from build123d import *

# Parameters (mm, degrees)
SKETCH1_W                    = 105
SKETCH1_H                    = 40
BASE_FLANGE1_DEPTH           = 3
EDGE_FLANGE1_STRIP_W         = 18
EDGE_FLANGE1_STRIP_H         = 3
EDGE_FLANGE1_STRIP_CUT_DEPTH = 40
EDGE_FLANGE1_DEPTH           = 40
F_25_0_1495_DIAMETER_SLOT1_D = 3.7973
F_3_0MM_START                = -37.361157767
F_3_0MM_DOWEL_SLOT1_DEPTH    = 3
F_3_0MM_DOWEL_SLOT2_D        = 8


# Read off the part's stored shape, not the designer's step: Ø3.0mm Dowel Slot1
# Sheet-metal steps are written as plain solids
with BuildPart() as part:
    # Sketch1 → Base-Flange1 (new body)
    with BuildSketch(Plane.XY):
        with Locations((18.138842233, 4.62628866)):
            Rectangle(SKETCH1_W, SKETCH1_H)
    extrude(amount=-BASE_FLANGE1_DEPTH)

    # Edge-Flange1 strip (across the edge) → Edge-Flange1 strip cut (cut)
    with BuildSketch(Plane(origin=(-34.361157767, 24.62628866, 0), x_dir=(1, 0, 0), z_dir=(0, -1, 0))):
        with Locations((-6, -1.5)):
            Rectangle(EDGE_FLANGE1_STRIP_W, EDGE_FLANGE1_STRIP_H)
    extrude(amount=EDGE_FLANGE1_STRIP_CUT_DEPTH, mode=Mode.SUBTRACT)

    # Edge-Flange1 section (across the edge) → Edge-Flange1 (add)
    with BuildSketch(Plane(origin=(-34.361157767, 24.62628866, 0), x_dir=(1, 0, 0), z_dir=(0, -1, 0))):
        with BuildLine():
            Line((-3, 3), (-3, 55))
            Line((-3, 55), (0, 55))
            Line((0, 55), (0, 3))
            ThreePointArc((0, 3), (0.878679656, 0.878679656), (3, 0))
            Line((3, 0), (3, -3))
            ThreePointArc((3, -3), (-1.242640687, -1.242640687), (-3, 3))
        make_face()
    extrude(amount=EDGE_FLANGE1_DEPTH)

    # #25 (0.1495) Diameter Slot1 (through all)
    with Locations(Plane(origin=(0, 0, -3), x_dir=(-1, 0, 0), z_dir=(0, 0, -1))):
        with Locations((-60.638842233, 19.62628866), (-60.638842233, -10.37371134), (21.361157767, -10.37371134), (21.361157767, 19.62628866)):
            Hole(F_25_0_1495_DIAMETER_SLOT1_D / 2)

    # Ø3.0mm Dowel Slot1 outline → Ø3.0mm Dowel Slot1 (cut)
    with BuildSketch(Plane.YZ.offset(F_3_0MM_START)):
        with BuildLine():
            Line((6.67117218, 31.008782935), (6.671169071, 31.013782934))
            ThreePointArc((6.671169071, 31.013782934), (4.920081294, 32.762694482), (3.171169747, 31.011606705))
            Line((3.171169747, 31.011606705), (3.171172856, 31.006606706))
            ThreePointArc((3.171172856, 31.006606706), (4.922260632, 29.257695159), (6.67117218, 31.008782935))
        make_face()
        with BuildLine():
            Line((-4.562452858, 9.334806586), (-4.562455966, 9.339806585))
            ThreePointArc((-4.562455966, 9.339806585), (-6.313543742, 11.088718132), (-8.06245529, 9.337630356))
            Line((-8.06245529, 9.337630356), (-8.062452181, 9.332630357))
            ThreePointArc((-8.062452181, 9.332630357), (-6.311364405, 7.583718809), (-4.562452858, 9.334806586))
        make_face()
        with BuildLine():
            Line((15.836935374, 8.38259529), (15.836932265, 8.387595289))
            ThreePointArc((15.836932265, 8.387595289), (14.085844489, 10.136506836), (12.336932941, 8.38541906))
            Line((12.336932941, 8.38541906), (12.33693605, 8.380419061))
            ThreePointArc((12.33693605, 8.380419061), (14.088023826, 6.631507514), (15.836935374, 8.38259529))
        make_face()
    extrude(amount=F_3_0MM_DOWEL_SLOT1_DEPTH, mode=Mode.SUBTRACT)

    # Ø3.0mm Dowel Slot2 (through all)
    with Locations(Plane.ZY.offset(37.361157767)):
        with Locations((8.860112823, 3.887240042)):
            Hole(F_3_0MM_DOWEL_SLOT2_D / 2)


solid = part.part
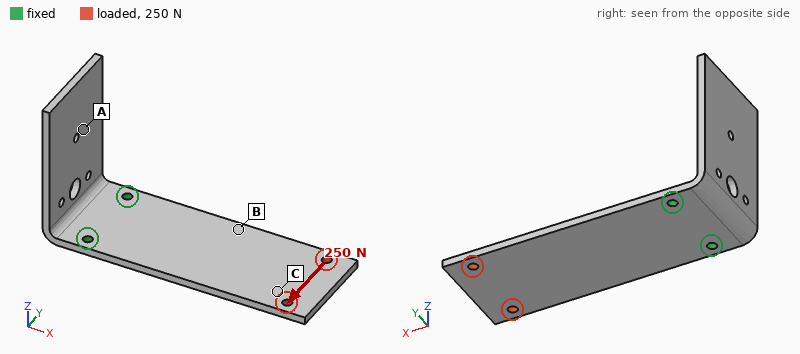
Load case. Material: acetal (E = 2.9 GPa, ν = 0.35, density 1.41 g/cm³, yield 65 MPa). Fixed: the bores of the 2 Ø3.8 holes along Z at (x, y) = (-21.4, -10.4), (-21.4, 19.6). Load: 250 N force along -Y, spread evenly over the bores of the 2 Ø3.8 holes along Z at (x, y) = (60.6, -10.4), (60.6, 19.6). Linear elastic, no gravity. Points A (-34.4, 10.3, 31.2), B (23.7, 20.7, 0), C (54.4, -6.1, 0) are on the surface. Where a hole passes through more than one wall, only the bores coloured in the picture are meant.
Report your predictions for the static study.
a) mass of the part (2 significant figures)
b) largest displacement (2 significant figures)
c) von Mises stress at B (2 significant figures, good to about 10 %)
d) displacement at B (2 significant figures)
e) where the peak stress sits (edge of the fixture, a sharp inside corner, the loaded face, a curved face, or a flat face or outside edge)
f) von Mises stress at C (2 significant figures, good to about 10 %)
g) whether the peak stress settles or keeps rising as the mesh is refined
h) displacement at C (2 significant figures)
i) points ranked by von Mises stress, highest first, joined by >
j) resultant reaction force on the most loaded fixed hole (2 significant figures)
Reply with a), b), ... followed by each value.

a) 27 g
b) 1.4 mm
c) 9.4 MPa
d) 0.54 mm
e) edge of the fixture
f) 4.7 MPa
g) keeps rising
h) 1.1 mm
i) B > C > A
j) 670 N
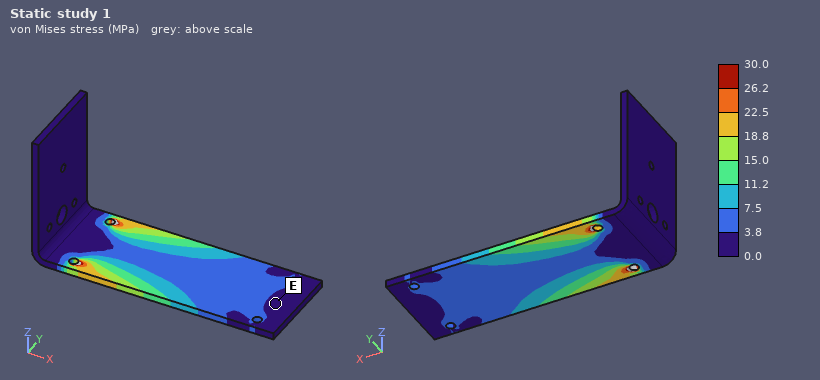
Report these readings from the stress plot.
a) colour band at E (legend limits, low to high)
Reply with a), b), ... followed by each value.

a) 0.0 to 3.8 MPa
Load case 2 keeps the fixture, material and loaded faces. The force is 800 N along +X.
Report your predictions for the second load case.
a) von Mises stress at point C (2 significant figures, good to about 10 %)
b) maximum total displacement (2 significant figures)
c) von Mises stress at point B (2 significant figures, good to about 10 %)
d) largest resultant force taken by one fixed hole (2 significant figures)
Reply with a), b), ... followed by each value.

a) 7.8 MPa
b) 0.23 mm
c) 6.7 MPa
d) 400 N
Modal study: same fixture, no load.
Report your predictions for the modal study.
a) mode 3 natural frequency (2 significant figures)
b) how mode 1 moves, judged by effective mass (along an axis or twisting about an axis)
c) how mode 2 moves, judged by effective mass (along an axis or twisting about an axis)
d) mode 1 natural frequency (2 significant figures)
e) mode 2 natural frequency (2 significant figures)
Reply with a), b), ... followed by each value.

a) 400 Hz
b) along Z
c) along X
d) 83 Hz
e) 150 Hz
